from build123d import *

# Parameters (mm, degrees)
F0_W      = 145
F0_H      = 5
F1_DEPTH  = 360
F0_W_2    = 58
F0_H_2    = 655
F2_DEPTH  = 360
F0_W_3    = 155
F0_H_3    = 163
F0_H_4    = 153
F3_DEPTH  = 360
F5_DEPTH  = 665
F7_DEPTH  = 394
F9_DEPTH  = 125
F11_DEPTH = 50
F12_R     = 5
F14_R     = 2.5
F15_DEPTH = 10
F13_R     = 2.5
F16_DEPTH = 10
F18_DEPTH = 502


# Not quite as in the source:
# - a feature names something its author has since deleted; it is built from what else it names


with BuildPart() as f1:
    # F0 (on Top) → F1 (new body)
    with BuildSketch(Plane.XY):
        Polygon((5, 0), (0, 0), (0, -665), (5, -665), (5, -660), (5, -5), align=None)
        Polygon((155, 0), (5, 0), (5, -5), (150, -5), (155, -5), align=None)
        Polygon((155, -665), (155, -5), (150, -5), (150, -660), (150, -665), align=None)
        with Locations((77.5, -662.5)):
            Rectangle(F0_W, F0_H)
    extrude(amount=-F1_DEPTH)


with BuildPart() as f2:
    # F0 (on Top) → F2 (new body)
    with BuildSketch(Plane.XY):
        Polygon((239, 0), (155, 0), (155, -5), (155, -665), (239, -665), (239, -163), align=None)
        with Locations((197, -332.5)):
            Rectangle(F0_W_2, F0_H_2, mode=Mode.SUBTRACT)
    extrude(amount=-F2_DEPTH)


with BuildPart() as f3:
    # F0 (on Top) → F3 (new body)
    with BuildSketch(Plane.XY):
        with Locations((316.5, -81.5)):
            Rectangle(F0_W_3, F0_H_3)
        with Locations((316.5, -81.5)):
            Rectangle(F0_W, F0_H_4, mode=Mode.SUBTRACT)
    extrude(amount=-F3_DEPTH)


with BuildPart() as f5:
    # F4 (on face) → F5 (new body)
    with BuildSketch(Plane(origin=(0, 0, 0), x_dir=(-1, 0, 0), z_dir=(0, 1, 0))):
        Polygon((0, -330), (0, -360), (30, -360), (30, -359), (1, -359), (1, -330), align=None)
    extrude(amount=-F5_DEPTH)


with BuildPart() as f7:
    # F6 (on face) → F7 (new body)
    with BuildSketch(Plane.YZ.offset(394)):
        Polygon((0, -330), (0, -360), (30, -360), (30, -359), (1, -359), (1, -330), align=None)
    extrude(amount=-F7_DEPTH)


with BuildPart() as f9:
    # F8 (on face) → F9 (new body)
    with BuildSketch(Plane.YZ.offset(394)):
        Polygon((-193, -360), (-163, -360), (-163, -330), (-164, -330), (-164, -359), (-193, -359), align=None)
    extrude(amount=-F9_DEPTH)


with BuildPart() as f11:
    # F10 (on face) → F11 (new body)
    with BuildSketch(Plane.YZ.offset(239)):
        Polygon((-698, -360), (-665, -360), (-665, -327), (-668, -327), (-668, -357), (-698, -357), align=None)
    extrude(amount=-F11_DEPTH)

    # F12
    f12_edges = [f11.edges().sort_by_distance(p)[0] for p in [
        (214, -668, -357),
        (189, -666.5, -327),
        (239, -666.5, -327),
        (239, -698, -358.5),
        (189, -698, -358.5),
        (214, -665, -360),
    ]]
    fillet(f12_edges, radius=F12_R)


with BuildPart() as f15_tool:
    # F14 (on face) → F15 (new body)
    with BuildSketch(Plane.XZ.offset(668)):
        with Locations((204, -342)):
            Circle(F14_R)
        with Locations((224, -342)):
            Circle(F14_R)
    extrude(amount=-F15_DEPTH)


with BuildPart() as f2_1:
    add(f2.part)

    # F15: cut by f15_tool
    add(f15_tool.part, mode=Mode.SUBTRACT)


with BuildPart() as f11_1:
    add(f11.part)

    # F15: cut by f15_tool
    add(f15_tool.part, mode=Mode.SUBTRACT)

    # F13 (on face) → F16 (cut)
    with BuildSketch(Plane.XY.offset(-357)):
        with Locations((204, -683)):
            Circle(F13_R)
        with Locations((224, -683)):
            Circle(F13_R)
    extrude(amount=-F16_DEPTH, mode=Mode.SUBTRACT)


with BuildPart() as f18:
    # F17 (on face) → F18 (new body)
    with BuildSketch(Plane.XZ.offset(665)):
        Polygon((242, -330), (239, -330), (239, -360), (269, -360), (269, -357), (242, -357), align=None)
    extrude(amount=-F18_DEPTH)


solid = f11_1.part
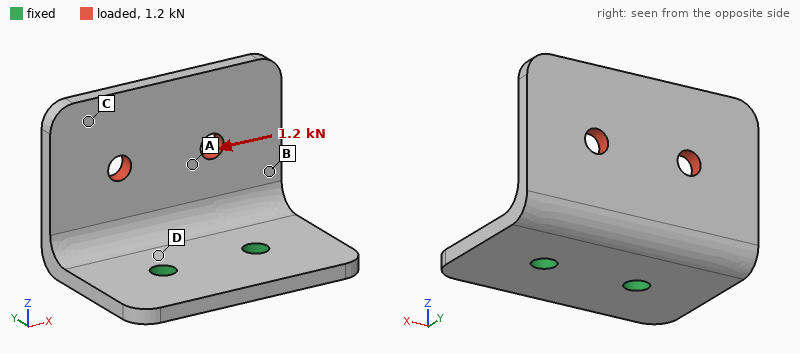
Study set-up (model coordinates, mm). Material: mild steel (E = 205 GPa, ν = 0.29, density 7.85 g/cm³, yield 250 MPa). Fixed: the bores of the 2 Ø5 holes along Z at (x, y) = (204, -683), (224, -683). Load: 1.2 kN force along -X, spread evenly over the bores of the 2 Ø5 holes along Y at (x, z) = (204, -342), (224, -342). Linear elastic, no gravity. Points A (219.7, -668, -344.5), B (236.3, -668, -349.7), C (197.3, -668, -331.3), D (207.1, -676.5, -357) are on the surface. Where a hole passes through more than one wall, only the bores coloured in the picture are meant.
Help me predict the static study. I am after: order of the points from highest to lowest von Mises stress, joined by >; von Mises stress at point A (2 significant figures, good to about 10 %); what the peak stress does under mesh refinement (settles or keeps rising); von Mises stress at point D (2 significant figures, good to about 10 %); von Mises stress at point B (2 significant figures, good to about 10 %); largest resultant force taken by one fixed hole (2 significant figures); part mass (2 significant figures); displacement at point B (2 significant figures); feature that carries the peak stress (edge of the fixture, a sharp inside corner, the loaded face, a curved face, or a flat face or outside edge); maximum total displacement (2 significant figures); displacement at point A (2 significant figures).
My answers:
D > B > A > C
45 MPa
keeps rising
110 MPa
59 MPa
1.2 kN
72 g
0.065 mm
edge of the fixture
0.11 mm
0.045 mm
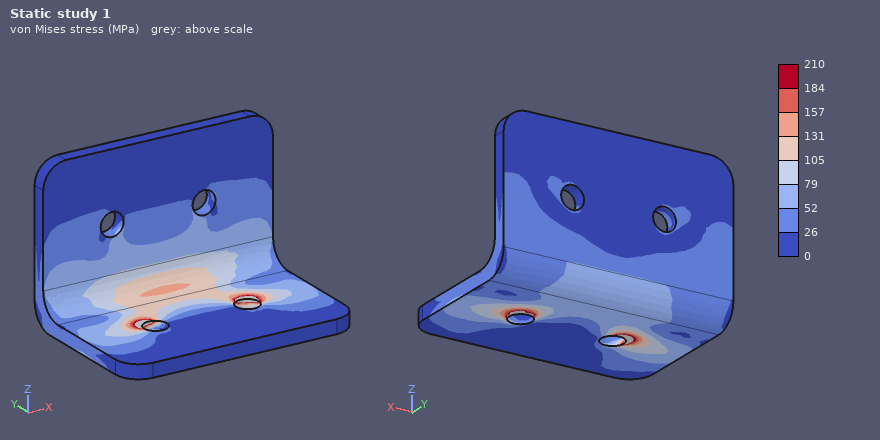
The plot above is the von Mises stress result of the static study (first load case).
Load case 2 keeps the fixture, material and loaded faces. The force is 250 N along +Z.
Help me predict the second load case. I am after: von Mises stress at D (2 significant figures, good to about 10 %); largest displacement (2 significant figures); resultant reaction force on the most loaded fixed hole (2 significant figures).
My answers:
35 MPa
45 µm
130 N
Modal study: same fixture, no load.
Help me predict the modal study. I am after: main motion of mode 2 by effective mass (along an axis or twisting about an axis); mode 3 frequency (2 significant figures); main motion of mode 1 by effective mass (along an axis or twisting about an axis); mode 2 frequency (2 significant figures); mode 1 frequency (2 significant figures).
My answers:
along X
4800 Hz
along Y
2700 Hz
1600 Hz
